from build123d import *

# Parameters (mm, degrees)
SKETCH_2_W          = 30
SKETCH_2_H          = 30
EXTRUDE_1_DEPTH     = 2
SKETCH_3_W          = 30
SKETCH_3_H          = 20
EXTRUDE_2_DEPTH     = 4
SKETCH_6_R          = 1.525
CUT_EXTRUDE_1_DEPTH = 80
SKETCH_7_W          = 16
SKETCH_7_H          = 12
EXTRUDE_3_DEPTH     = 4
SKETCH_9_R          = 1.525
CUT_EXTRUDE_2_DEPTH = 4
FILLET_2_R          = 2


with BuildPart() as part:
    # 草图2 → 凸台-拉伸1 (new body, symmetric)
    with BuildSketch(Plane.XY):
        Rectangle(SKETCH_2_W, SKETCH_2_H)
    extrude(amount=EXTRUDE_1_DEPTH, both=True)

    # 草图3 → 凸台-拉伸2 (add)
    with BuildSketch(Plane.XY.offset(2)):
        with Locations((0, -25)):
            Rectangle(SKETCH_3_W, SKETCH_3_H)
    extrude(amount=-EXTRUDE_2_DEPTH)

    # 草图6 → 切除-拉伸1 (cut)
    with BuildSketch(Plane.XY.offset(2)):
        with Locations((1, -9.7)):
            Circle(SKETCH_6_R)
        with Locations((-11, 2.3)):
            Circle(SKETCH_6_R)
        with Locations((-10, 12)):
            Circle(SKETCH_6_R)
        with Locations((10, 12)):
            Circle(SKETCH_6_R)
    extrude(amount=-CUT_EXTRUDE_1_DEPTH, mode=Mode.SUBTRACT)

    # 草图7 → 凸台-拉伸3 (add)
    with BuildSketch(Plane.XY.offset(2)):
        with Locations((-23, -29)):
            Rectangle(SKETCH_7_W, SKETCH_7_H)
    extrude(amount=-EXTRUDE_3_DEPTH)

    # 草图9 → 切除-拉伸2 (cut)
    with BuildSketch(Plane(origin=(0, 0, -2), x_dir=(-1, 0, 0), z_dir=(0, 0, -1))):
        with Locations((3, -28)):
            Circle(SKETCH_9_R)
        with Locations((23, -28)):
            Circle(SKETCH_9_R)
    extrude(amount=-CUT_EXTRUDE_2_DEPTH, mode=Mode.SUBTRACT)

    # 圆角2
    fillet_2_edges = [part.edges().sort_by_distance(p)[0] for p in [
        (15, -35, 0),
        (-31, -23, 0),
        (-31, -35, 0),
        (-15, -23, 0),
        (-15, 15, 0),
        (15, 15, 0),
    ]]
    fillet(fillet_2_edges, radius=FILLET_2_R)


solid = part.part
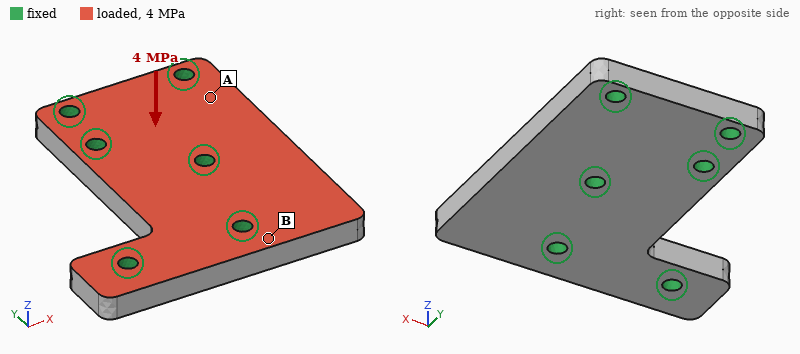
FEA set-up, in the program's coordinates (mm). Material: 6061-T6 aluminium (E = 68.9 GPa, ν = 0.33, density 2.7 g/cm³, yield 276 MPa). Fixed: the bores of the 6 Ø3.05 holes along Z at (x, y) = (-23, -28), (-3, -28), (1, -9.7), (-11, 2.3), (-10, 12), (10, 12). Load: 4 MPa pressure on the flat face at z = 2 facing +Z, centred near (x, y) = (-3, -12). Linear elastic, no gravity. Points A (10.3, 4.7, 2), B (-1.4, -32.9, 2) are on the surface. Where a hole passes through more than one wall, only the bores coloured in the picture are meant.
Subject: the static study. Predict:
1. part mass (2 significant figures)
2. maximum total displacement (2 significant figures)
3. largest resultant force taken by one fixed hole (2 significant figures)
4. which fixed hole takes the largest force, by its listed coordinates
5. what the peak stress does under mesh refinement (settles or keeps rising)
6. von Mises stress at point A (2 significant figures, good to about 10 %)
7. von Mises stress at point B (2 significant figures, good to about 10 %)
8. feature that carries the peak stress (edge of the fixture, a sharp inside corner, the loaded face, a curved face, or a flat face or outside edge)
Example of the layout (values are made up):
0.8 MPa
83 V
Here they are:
18 g
0.12 mm
2.0 kN
(1, -9.7)
keeps rising
42 MPa
100 MPa
edge of the fixture
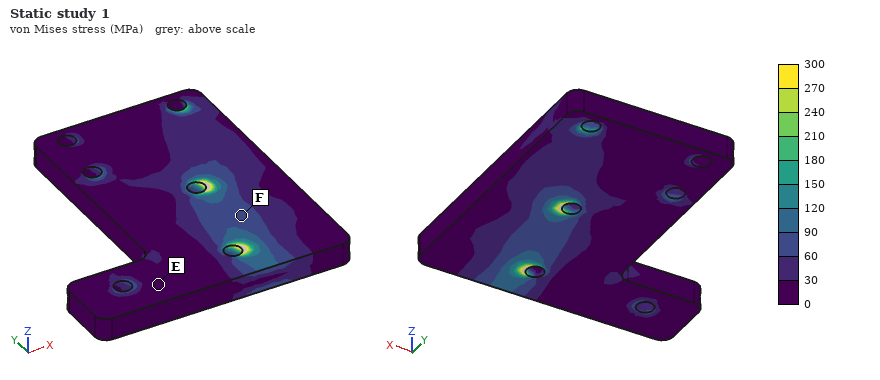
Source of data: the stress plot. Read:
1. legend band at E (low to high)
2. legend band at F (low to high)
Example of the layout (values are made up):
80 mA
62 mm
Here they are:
0 to 30 MPa
60 to 90 MPa
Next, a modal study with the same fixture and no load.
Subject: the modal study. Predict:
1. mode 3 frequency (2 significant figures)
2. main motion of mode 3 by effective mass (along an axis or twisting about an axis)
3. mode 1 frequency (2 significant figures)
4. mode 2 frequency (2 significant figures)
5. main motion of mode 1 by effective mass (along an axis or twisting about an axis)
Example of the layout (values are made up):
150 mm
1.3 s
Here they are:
26 kHz
along Z
12 kHz
21 kHz
along Z
